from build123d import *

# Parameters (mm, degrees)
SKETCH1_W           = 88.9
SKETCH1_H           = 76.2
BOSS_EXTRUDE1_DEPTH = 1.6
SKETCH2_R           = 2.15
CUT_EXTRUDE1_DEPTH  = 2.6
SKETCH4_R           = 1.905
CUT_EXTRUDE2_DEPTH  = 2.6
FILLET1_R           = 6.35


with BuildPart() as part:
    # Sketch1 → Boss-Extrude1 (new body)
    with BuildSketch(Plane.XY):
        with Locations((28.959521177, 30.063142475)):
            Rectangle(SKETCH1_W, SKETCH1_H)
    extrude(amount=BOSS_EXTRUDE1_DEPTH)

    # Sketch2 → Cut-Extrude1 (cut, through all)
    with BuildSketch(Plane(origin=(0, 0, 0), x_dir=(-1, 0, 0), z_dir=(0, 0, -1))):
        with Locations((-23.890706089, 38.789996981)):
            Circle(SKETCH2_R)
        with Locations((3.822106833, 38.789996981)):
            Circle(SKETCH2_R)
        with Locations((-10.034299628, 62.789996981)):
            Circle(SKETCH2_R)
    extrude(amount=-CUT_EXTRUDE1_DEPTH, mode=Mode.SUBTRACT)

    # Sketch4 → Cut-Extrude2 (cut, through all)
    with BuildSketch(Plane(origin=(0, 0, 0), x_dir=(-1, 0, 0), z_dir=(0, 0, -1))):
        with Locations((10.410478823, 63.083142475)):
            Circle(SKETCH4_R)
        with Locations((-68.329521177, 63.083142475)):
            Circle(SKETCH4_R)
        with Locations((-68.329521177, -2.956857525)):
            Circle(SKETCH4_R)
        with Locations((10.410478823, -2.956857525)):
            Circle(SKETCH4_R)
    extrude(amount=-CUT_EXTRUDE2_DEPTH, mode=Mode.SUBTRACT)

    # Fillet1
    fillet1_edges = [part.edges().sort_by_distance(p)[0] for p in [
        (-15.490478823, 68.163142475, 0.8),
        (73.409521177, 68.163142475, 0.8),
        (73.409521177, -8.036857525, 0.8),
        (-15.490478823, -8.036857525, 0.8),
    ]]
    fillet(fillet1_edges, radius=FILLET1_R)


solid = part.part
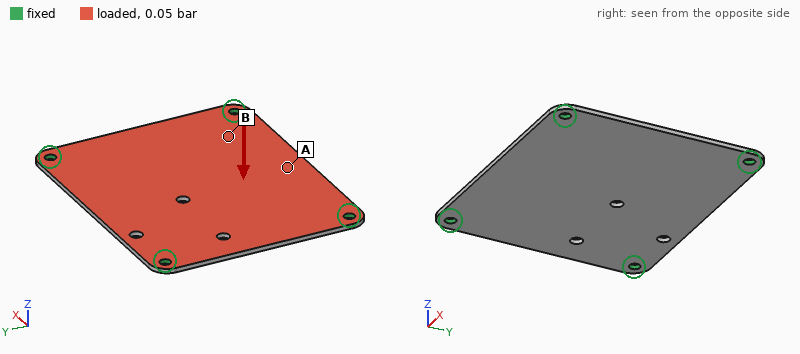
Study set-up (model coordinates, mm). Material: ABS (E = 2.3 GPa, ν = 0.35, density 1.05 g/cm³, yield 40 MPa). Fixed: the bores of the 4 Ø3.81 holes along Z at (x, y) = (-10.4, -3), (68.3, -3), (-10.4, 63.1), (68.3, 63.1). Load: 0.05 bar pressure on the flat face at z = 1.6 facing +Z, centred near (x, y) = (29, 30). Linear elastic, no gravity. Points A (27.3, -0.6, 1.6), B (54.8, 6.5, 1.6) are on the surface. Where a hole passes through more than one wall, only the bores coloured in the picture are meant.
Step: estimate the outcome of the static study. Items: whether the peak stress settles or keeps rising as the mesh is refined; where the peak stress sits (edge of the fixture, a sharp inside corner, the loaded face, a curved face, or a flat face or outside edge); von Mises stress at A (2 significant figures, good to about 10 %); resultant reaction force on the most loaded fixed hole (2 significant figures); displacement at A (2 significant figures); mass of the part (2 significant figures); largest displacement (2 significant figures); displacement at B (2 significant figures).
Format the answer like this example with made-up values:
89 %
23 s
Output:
keeps rising
edge of the fixture
3.8 MPa
8.4 N
0.89 mm
11 g
1.2 mm
0.46 mm
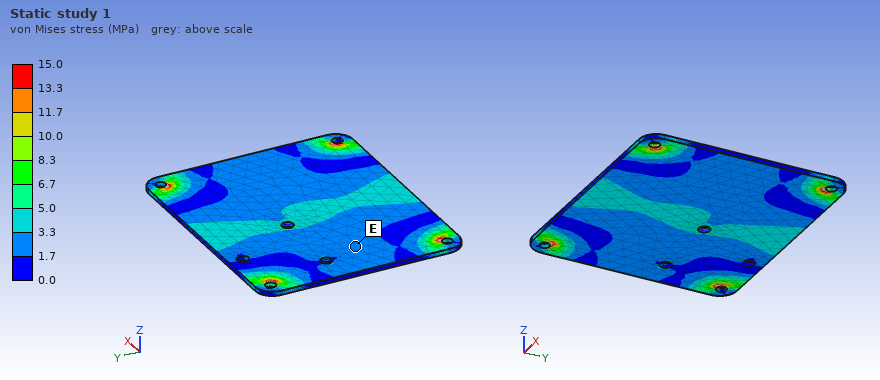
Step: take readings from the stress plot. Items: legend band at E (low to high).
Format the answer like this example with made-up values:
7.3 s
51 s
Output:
1.7 to 3.3 MPa
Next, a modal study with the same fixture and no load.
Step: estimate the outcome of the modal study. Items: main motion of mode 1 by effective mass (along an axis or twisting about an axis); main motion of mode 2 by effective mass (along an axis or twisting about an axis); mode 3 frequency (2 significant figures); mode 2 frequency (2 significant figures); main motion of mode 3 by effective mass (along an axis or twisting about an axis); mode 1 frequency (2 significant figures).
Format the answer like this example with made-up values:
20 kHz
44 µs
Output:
along Z
twisting about X
600 Hz
480 Hz
twisting about Y
300 Hz
